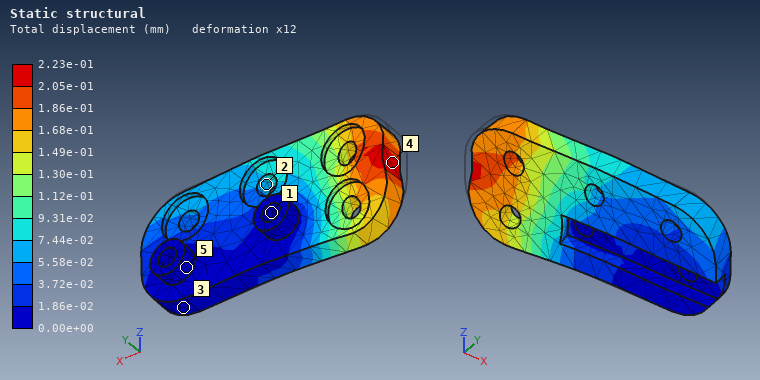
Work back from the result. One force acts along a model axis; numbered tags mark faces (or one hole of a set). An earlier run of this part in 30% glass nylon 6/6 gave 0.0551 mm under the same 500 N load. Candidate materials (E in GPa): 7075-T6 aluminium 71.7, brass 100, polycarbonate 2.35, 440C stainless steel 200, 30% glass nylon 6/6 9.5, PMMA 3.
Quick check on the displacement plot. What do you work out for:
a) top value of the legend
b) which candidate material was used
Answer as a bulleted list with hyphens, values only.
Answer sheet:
- 2.23e-01 mm
- polycarbonate
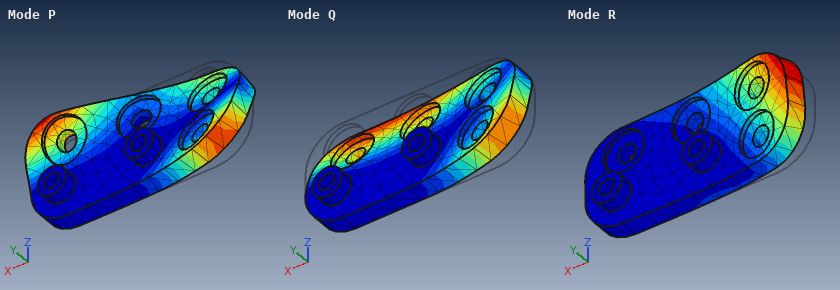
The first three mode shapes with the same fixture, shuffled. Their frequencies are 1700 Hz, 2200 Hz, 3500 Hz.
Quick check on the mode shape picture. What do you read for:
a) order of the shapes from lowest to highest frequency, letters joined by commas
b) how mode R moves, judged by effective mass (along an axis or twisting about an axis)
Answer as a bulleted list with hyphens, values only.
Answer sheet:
- R, Q, P
- along Y
